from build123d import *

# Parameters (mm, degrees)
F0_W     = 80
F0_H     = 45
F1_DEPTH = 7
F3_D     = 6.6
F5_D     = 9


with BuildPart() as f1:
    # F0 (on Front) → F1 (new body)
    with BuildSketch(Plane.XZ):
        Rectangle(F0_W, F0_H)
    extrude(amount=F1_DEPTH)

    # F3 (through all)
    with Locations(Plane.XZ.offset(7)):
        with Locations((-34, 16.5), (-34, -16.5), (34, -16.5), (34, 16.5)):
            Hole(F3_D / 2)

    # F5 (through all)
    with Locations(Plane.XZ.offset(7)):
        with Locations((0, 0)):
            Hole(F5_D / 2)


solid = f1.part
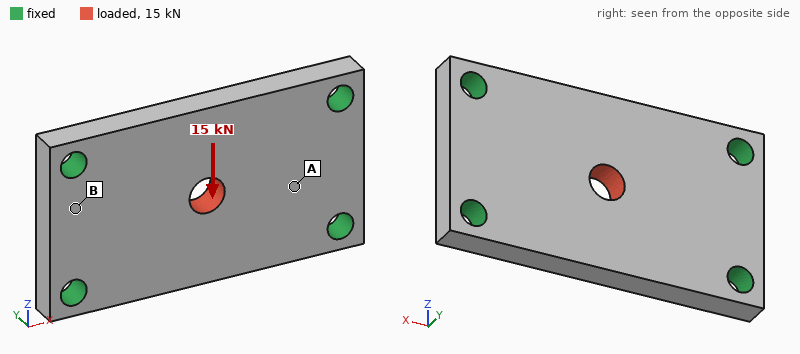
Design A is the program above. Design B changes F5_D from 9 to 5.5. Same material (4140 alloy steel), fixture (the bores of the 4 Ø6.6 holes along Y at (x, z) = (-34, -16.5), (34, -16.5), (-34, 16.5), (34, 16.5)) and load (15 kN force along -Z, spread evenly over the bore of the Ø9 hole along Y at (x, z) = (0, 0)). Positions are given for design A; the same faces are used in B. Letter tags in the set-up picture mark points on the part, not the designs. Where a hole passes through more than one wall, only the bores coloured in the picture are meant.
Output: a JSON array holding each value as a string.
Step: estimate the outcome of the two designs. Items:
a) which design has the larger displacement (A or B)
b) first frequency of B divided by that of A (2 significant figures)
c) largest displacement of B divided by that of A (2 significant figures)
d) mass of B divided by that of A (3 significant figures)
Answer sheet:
["B", "1.00", "1.1", "1.01"]
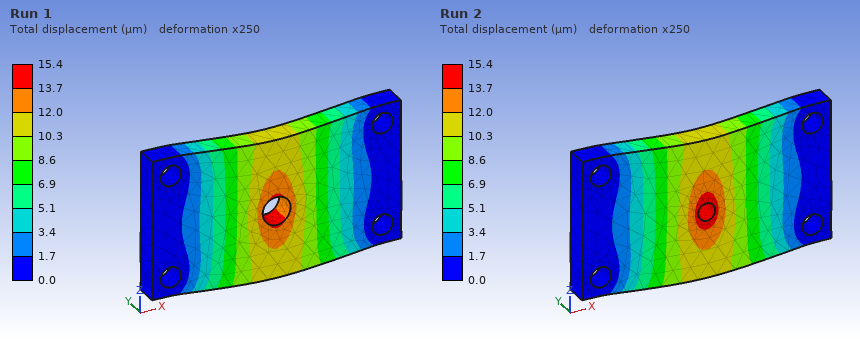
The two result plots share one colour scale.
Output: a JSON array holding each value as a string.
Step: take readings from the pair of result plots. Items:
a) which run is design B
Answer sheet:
["Run 2"]
